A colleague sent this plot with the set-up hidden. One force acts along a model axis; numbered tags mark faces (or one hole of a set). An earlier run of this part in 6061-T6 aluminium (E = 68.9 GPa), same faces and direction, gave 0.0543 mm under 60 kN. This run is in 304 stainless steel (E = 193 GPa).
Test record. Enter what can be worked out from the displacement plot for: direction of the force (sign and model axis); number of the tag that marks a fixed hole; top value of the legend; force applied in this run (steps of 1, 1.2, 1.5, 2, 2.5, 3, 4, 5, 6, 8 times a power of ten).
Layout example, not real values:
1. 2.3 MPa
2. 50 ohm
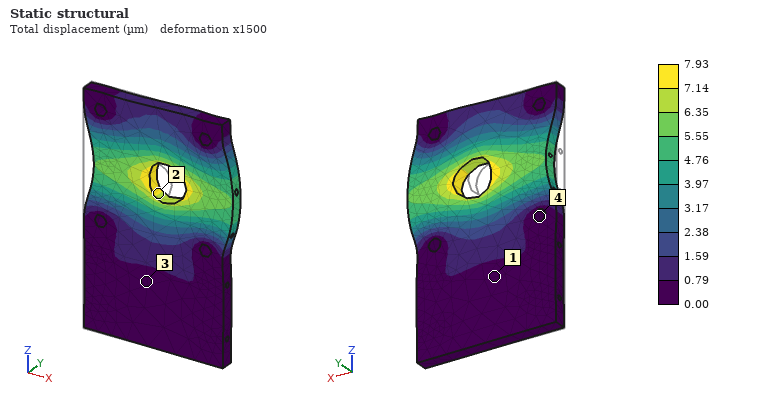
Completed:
1. +X
2. 4
3. 7.93 µm
4. 25 kN
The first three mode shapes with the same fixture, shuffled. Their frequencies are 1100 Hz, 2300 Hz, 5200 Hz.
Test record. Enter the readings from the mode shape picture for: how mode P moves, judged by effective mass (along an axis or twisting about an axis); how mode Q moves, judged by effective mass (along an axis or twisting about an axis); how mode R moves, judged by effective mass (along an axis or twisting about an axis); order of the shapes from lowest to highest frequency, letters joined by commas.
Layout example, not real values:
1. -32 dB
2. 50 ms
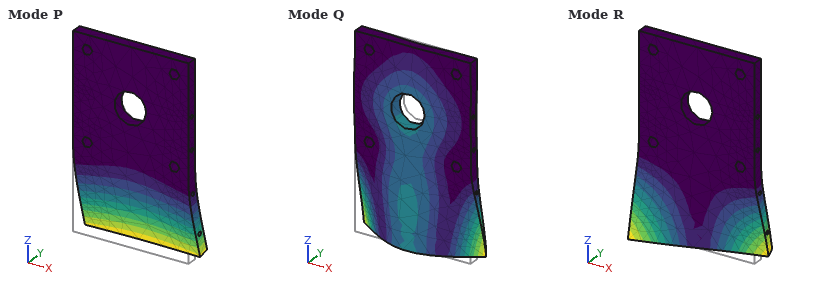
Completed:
1. along Y
2. along Y
3. twisting about Z
4. P, R, Q
